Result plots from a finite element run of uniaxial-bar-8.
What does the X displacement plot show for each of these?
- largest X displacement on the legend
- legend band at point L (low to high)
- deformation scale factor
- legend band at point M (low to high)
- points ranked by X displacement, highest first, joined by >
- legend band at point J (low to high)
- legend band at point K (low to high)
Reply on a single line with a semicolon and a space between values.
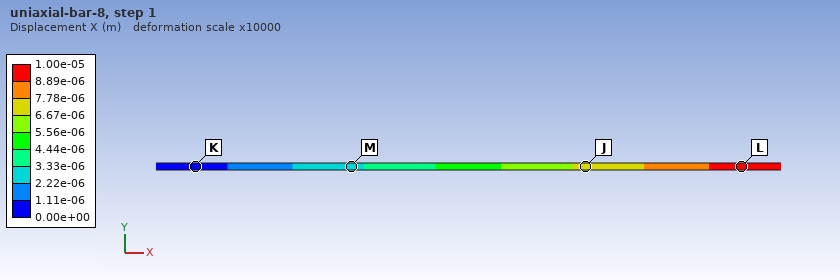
1.00e-05 m; 8.89e-06 to 1.00e-05 m; 10000; 2.22e-06 to 3.33e-06 m; L > J > M > K; 6.67e-06 to 7.78e-06 m; 0.00e+00 to 1.11e-06 m
